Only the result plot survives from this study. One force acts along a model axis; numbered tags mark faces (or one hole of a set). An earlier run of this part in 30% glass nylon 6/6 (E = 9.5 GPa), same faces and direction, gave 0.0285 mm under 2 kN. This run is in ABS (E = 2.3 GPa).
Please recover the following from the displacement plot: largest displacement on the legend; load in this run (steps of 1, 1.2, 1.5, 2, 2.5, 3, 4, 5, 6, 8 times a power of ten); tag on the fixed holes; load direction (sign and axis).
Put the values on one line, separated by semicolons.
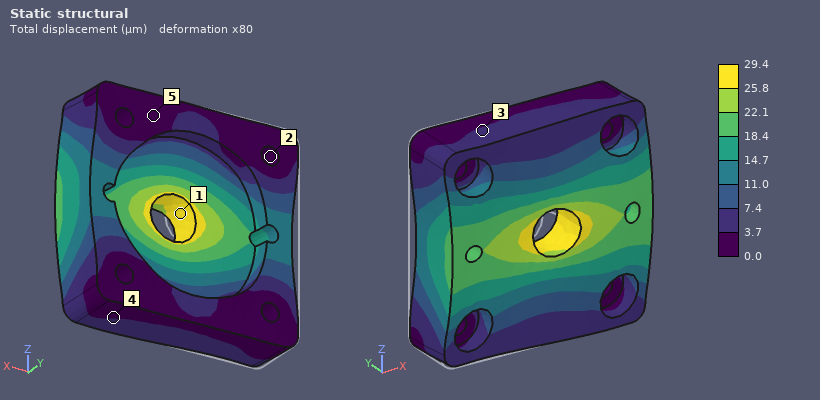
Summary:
29.4 µm; 500 N; 2; +X
